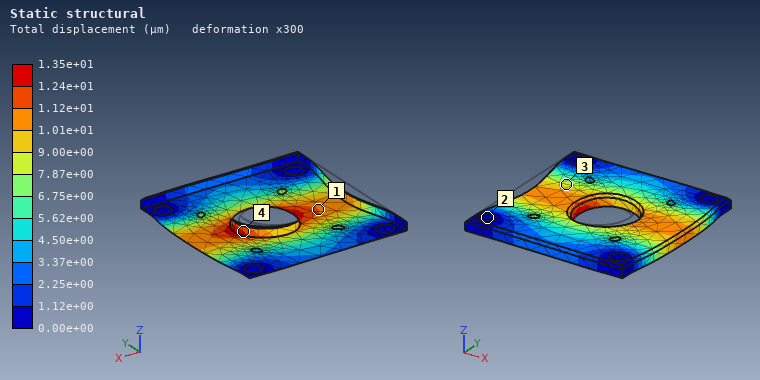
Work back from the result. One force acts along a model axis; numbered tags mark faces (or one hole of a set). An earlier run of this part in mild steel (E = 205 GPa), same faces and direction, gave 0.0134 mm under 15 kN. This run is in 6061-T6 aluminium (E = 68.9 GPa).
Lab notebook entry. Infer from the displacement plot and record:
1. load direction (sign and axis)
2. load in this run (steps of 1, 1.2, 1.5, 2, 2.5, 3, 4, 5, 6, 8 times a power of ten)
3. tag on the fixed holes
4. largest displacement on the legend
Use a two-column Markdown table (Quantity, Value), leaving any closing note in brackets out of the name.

| Quantity | Value |
|---|---|
| load direction | +X |
| load in this run | 5 kN |
| tag on the fixed holes | 2 |
| largest displacement on the legend | 1.35e+01 µm |
